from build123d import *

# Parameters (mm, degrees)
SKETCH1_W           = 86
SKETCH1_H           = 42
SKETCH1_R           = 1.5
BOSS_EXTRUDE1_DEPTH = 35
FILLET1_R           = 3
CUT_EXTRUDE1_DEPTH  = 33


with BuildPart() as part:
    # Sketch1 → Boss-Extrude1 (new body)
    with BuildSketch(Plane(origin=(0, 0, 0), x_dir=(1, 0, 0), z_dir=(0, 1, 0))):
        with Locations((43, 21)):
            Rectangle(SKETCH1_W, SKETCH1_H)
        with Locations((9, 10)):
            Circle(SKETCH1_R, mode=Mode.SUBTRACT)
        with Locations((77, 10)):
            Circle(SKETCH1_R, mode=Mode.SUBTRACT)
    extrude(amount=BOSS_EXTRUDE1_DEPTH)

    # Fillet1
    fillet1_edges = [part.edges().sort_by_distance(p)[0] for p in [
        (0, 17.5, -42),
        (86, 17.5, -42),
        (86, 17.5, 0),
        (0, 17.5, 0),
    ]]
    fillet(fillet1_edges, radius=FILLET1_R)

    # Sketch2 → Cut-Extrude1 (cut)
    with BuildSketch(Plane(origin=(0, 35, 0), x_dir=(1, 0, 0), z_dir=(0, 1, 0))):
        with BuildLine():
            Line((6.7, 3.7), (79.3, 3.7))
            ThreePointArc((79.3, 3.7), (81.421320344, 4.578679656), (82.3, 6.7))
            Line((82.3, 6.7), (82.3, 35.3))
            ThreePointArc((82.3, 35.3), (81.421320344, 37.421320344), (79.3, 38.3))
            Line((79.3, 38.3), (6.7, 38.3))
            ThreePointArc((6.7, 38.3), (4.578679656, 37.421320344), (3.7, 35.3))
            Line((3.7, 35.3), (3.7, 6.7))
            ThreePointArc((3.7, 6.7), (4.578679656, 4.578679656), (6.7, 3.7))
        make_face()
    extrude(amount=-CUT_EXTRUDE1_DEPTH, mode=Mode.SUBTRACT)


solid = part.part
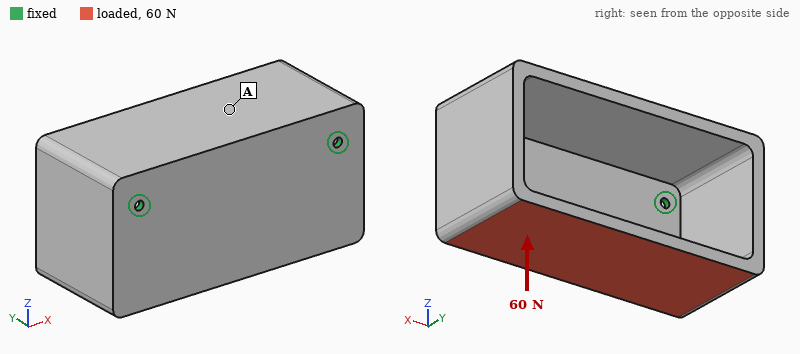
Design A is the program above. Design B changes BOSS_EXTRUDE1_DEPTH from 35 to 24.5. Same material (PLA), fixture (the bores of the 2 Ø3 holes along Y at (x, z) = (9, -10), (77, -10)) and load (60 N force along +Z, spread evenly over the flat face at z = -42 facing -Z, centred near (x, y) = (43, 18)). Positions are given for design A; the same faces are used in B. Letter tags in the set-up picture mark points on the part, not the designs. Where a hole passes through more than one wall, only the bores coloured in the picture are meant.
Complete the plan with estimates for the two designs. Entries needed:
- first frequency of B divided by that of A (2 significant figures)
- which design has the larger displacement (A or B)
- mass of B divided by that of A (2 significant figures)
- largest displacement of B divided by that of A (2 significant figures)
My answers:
1.3
A
0.74
0.62
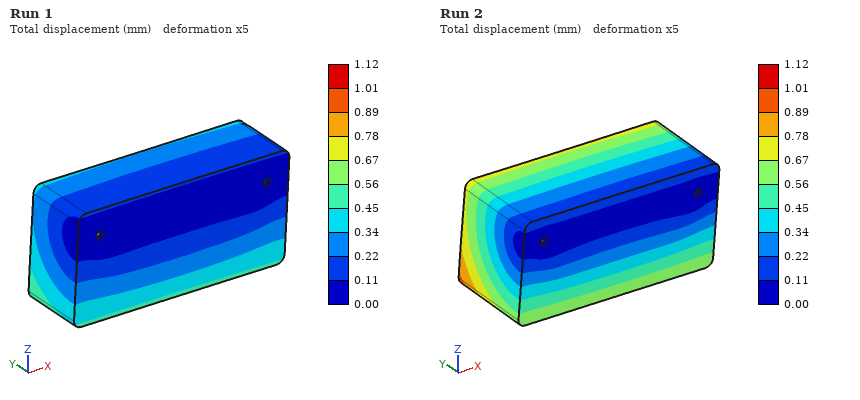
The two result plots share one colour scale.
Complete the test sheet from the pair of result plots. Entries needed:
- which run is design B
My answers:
Run 1
